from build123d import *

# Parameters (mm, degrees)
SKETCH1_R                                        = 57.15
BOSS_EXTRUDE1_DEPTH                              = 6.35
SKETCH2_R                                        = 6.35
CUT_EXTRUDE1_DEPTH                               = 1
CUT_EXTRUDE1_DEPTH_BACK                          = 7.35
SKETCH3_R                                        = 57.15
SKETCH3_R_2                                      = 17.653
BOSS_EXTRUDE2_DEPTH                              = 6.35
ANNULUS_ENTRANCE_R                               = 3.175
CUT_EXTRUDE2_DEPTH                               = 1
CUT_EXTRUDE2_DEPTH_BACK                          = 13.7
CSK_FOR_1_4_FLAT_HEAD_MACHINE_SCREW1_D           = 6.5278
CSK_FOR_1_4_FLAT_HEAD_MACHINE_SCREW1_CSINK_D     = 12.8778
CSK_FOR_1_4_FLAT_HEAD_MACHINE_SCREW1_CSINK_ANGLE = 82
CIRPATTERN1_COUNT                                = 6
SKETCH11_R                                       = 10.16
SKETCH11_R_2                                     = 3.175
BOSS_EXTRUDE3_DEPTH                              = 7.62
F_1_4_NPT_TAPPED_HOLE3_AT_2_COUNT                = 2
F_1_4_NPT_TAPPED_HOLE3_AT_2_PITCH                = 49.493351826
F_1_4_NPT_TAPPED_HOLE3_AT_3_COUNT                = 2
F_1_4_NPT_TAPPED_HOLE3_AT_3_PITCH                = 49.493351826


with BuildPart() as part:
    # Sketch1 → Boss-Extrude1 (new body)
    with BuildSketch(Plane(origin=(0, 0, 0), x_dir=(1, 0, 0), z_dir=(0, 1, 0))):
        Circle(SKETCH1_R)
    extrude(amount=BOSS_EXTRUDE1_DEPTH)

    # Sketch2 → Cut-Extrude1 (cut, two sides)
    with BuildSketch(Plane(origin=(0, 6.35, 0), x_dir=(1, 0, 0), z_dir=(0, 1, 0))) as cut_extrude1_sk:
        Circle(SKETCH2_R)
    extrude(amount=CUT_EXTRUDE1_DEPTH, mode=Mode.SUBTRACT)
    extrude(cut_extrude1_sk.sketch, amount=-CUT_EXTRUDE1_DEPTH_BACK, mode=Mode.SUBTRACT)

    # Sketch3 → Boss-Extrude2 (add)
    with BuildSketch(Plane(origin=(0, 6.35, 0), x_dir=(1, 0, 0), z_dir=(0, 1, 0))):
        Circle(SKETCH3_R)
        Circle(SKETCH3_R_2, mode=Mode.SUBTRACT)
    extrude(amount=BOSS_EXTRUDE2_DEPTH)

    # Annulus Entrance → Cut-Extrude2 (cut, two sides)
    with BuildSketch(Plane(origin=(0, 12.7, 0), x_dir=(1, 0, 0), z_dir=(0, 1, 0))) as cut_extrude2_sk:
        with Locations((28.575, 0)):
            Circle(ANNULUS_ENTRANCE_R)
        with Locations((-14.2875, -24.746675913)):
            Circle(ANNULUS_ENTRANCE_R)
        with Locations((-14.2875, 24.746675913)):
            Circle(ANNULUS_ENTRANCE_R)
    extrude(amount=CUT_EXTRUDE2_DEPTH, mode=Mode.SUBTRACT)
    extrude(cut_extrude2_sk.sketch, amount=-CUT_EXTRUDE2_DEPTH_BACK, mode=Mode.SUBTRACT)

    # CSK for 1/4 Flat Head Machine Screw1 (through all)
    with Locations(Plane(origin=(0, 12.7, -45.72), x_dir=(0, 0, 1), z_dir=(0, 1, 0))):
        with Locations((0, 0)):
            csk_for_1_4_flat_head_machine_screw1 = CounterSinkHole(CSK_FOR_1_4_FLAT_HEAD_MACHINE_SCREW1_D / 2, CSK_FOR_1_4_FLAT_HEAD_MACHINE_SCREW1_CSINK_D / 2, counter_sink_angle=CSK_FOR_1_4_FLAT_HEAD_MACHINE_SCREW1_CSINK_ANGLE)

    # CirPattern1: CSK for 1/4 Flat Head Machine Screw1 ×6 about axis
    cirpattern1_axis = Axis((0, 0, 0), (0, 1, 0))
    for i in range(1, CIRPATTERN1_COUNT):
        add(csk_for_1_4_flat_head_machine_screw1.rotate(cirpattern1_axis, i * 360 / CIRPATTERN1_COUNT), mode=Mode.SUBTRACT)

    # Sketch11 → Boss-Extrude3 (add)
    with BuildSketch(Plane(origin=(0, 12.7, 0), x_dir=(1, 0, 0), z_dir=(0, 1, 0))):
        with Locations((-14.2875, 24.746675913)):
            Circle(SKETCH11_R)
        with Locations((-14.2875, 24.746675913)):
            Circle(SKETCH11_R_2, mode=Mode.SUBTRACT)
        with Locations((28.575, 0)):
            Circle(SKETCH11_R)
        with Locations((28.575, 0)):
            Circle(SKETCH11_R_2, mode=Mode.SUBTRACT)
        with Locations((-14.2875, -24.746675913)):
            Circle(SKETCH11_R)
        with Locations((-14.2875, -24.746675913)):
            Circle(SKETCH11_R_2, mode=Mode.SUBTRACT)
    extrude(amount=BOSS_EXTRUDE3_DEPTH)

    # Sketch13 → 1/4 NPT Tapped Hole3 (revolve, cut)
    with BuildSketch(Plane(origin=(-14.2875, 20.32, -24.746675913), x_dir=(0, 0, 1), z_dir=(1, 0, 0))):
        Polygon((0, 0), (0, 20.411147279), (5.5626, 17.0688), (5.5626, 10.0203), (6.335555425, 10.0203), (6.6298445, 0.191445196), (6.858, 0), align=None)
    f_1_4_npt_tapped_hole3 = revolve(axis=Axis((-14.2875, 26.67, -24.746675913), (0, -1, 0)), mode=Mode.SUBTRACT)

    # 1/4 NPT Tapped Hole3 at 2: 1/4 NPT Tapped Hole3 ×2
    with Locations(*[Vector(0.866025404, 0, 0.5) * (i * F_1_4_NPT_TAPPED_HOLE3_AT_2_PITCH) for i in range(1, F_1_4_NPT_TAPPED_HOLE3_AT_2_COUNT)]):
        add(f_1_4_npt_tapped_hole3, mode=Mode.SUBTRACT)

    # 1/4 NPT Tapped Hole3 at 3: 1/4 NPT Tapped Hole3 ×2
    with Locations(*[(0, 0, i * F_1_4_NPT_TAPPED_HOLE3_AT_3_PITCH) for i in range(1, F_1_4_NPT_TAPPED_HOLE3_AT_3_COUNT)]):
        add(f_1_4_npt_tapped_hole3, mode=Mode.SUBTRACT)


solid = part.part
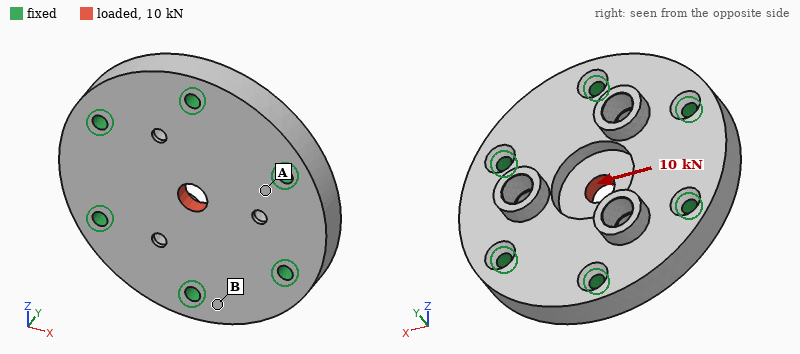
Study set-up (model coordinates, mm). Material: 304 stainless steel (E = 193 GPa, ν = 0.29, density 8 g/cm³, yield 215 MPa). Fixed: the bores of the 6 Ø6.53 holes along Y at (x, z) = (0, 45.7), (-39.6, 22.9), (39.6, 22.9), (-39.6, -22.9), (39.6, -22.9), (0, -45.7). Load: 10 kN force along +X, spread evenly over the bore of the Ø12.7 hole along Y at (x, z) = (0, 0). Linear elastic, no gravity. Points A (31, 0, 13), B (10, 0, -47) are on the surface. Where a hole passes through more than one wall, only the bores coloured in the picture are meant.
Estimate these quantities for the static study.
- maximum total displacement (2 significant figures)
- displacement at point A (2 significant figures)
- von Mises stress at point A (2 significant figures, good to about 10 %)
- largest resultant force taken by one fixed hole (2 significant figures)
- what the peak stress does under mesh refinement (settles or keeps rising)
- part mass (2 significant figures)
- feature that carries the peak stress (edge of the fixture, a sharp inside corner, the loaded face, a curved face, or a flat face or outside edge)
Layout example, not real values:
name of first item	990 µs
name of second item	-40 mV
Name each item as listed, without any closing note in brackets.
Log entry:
maximum total displacement	4.2 µm
displacement at point A	0.78 µm
von Mises stress at point A	14 MPa
largest resultant force taken by one fixed hole	2.3 kN
what the peak stress does under mesh refinement	keeps rising
part mass	970 g
feature that carries the peak stress	a sharp inside corner
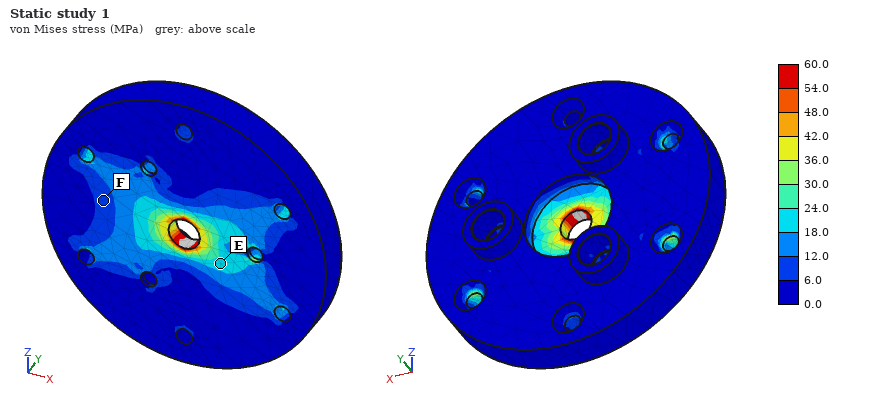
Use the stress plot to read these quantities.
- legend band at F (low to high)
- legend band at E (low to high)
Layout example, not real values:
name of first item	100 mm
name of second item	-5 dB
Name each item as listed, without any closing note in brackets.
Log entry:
legend band at F	6.0 to 12.0 MPa
legend band at E	18.0 to 24.0 MPa
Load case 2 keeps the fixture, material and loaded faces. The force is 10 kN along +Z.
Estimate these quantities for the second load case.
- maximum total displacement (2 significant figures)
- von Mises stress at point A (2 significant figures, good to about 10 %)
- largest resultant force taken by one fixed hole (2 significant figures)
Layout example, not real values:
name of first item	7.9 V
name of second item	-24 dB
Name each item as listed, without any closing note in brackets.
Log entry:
maximum total displacement	4.2 µm
von Mises stress at point A	7.2 MPa
largest resultant force taken by one fixed hole	2.5 kN
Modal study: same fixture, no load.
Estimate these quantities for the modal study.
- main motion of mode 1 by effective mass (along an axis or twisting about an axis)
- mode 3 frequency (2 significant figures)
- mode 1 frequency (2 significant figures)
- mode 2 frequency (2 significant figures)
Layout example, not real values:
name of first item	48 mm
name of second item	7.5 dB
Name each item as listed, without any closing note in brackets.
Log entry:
main motion of mode 1 by effective mass	along Y
mode 3 frequency	16 kHz
mode 1 frequency	9400 Hz
mode 2 frequency	15 kHz
